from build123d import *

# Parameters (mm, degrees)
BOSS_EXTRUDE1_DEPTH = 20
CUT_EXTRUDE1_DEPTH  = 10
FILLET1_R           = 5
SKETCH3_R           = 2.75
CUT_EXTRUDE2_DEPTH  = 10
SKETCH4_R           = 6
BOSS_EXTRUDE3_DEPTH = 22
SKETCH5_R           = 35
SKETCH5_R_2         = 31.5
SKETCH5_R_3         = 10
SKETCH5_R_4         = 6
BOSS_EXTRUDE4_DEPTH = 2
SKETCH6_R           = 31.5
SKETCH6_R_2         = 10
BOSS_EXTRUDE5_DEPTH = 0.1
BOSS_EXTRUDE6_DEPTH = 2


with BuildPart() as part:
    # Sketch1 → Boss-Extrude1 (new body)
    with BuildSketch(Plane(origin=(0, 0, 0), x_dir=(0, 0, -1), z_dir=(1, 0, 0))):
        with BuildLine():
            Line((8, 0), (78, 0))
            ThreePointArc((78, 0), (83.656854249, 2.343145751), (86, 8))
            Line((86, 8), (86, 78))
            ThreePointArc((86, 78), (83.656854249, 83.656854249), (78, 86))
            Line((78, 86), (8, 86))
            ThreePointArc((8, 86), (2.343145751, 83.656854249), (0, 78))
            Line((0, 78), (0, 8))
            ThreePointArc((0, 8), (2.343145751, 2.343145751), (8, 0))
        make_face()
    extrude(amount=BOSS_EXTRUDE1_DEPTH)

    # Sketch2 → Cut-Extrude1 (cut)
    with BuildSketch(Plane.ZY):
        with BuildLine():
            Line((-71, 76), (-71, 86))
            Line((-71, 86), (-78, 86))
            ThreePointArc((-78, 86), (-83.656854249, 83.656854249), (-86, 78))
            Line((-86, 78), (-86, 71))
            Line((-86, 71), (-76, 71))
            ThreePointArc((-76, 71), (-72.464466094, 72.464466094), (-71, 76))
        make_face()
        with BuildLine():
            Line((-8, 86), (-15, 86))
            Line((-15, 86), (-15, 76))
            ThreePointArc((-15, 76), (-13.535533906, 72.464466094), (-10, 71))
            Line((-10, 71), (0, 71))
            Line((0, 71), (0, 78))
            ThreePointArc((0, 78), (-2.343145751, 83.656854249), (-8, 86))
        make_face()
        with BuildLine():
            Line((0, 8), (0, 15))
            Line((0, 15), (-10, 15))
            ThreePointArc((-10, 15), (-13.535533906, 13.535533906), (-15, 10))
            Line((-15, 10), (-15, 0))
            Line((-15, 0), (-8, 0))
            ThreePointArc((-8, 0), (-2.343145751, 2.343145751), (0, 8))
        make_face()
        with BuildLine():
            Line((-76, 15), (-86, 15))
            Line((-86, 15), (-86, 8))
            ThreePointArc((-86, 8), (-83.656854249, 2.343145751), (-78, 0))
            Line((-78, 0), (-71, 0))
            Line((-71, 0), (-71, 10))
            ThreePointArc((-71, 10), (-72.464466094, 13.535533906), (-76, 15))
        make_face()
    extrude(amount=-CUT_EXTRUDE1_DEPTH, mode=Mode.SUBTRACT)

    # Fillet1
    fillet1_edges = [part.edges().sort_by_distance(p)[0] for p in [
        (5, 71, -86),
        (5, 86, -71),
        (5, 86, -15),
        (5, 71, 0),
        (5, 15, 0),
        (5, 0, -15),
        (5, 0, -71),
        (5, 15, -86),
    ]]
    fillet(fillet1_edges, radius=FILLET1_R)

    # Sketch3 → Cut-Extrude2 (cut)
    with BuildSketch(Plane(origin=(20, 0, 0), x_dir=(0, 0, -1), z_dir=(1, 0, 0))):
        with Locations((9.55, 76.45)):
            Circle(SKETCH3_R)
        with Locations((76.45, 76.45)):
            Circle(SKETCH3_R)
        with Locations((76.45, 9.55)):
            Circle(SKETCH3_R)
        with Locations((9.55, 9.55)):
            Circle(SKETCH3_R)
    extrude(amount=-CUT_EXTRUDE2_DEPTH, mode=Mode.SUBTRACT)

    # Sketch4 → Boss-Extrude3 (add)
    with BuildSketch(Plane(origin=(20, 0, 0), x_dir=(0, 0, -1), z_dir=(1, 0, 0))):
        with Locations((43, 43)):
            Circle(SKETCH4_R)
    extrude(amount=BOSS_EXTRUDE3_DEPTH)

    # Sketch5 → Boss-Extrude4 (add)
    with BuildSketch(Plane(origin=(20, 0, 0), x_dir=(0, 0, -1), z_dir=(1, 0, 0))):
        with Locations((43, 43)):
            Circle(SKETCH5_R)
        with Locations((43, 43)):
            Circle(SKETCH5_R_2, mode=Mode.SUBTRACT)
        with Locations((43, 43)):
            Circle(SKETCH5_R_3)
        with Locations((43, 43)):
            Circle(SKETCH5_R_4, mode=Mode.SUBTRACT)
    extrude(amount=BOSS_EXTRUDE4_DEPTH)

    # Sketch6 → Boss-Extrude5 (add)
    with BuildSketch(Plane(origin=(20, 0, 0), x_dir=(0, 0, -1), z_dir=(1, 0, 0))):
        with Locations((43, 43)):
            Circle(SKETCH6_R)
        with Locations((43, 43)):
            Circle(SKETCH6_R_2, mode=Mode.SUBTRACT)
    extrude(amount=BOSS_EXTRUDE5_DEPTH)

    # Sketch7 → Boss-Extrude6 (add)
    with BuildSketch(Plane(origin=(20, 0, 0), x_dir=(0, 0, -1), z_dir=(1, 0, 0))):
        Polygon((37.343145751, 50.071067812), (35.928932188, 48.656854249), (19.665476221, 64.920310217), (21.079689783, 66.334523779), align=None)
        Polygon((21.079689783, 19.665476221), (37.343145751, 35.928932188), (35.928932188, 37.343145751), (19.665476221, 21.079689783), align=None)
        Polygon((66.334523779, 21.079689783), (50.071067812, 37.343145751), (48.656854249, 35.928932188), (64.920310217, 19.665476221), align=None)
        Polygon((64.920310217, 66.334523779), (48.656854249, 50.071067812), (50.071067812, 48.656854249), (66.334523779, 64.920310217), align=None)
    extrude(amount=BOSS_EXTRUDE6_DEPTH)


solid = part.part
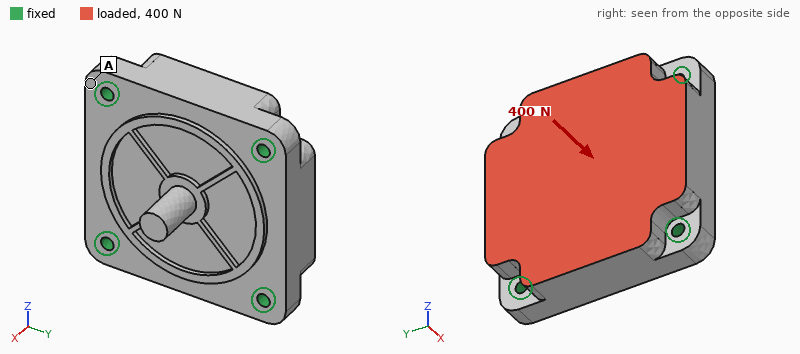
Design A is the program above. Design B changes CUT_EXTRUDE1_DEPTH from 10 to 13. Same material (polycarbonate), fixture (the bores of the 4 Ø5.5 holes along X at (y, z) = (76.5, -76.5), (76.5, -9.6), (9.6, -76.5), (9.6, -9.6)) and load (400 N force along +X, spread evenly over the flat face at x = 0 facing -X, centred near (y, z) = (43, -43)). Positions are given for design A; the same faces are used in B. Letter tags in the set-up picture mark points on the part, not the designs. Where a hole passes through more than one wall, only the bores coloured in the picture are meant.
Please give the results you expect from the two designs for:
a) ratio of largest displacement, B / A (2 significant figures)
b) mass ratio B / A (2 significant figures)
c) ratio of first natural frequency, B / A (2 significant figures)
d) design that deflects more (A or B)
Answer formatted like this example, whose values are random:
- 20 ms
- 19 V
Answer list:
- 1.2
- 0.98
- 0.92
- B
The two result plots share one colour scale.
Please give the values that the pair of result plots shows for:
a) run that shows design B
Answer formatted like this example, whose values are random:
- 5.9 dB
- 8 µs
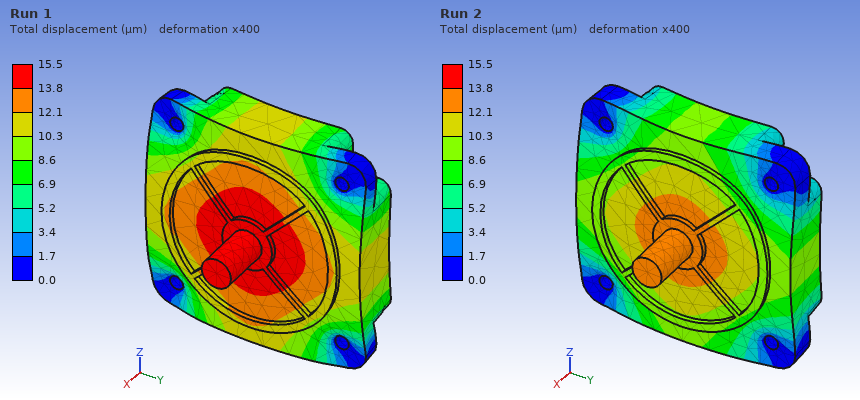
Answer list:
- Run 1
